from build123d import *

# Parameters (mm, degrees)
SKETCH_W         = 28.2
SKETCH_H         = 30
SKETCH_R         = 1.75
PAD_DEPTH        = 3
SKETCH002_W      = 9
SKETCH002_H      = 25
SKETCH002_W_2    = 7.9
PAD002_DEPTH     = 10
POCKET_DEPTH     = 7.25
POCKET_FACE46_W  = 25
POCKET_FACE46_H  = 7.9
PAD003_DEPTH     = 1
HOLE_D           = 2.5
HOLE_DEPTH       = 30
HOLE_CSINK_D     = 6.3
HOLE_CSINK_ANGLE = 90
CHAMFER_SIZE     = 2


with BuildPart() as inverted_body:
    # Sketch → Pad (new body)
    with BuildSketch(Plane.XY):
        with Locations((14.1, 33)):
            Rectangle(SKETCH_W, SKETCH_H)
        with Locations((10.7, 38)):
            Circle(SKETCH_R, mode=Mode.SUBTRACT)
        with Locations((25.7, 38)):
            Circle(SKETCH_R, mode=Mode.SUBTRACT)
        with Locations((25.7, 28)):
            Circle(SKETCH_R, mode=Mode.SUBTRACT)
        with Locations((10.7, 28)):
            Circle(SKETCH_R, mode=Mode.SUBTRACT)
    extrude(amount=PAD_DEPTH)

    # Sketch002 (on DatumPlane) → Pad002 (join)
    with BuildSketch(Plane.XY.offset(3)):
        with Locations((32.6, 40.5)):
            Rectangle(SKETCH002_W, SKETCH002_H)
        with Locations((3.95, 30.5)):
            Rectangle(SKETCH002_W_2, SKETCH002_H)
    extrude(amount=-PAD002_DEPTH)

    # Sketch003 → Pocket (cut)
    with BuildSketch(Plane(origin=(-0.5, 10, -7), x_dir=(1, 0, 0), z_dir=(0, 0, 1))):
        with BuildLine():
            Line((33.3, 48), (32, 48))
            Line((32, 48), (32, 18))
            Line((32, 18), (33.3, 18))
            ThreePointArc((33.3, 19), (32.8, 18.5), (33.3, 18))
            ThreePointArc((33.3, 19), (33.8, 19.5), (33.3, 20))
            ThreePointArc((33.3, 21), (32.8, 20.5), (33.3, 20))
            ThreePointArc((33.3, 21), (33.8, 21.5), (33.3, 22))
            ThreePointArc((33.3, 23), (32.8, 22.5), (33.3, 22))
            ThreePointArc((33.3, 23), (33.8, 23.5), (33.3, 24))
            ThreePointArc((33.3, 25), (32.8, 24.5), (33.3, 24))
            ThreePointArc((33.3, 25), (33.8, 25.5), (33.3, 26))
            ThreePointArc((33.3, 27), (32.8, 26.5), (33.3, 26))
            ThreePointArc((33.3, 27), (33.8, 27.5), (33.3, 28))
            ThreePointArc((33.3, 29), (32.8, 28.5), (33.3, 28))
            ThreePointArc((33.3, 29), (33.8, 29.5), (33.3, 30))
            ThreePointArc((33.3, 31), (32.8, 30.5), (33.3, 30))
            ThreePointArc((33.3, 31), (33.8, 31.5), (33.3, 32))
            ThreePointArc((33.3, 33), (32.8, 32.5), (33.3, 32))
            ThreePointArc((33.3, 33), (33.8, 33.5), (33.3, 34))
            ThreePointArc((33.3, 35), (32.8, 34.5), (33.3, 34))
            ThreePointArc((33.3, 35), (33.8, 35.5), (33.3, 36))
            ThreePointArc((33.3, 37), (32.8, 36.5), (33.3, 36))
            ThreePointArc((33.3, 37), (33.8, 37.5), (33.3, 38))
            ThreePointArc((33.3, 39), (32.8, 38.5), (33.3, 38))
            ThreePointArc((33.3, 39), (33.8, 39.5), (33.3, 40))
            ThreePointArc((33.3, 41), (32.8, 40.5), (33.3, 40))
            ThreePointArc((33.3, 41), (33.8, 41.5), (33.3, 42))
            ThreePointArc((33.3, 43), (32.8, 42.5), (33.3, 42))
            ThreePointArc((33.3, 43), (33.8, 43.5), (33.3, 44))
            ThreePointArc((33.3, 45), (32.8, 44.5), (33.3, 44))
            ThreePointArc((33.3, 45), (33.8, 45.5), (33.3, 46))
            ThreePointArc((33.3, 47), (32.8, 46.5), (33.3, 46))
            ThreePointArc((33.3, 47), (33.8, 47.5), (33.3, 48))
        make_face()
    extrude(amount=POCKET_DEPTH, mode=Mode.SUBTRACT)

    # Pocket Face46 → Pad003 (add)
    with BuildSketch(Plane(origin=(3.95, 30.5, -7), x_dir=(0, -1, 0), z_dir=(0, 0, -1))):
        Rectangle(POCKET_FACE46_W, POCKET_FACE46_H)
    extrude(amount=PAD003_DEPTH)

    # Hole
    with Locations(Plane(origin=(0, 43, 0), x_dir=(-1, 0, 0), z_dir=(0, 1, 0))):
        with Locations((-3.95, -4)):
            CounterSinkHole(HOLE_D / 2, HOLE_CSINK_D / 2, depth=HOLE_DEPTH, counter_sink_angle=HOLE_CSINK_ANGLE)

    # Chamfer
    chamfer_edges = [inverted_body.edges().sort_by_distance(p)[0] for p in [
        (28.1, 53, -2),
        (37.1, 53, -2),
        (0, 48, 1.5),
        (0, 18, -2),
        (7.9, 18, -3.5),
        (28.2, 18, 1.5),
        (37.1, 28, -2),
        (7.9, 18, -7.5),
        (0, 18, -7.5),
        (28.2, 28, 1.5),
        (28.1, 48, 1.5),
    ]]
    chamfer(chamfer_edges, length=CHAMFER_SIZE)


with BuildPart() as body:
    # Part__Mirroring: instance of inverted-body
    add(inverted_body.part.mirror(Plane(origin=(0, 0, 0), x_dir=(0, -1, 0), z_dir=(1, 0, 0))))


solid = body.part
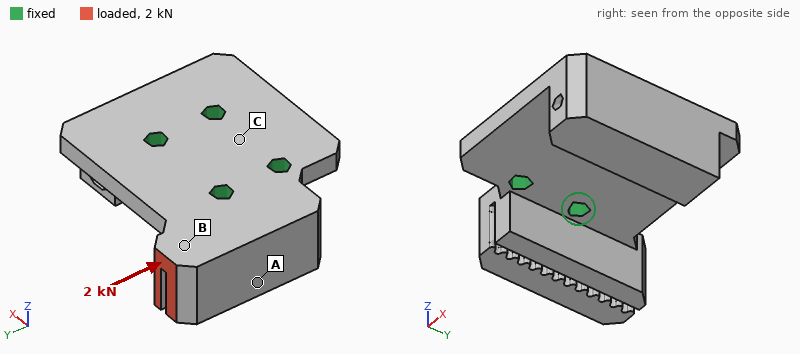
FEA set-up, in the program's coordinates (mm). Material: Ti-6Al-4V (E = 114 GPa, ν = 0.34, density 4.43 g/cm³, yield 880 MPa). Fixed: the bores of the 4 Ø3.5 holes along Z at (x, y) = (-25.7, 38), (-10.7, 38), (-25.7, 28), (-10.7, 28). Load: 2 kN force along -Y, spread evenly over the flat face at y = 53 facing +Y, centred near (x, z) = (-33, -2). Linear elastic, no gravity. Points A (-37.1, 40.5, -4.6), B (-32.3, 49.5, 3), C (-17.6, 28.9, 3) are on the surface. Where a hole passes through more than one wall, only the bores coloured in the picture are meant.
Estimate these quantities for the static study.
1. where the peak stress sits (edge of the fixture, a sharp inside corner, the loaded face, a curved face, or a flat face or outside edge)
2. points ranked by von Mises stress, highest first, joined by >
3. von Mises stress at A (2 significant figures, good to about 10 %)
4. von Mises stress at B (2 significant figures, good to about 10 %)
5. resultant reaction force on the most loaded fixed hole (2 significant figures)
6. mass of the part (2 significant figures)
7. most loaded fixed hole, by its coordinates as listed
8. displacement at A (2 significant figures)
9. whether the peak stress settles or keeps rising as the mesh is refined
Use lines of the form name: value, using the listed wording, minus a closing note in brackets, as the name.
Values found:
where the peak stress sits: edge of the fixture
points ranked by von Mises stress, highest first, joined by >: B > A > C
von Mises stress at A: 24 MPa
von Mises stress at B: 47 MPa
resultant reaction force on the most loaded fixed hole: 1.6 kN
mass of the part: 26 g
most loaded fixed hole, by its coordinates as listed: (-25.7, 38)
displacement at A: 18 µm
whether the peak stress settles or keeps rising as the mesh is refined: keeps rising
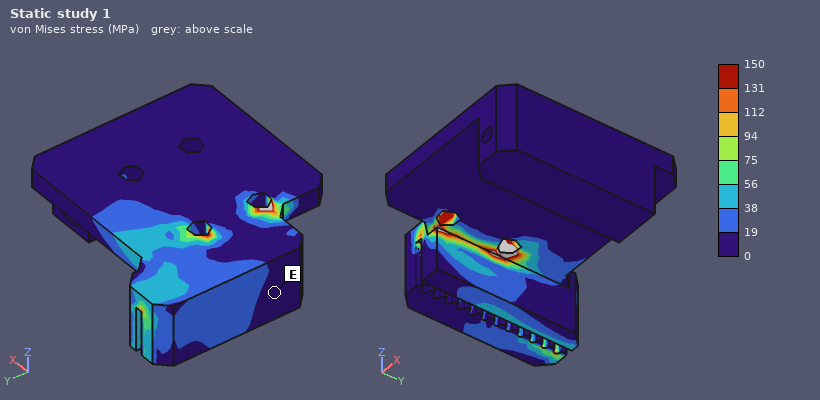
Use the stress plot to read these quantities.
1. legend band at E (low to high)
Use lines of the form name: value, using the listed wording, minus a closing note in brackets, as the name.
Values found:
legend band at E: 0 to 19 MPa
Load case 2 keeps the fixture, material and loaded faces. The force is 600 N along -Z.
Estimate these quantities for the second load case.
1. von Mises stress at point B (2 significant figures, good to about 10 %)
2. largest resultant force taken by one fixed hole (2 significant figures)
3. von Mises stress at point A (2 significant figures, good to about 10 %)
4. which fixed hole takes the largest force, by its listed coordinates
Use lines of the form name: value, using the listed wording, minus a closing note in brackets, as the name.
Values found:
von Mises stress at point B: 33 MPa
largest resultant force taken by one fixed hole: 1.3 kN
von Mises stress at point A: 27 MPa
which fixed hole takes the largest force, by its listed coordinates: (-25.7, 38)
